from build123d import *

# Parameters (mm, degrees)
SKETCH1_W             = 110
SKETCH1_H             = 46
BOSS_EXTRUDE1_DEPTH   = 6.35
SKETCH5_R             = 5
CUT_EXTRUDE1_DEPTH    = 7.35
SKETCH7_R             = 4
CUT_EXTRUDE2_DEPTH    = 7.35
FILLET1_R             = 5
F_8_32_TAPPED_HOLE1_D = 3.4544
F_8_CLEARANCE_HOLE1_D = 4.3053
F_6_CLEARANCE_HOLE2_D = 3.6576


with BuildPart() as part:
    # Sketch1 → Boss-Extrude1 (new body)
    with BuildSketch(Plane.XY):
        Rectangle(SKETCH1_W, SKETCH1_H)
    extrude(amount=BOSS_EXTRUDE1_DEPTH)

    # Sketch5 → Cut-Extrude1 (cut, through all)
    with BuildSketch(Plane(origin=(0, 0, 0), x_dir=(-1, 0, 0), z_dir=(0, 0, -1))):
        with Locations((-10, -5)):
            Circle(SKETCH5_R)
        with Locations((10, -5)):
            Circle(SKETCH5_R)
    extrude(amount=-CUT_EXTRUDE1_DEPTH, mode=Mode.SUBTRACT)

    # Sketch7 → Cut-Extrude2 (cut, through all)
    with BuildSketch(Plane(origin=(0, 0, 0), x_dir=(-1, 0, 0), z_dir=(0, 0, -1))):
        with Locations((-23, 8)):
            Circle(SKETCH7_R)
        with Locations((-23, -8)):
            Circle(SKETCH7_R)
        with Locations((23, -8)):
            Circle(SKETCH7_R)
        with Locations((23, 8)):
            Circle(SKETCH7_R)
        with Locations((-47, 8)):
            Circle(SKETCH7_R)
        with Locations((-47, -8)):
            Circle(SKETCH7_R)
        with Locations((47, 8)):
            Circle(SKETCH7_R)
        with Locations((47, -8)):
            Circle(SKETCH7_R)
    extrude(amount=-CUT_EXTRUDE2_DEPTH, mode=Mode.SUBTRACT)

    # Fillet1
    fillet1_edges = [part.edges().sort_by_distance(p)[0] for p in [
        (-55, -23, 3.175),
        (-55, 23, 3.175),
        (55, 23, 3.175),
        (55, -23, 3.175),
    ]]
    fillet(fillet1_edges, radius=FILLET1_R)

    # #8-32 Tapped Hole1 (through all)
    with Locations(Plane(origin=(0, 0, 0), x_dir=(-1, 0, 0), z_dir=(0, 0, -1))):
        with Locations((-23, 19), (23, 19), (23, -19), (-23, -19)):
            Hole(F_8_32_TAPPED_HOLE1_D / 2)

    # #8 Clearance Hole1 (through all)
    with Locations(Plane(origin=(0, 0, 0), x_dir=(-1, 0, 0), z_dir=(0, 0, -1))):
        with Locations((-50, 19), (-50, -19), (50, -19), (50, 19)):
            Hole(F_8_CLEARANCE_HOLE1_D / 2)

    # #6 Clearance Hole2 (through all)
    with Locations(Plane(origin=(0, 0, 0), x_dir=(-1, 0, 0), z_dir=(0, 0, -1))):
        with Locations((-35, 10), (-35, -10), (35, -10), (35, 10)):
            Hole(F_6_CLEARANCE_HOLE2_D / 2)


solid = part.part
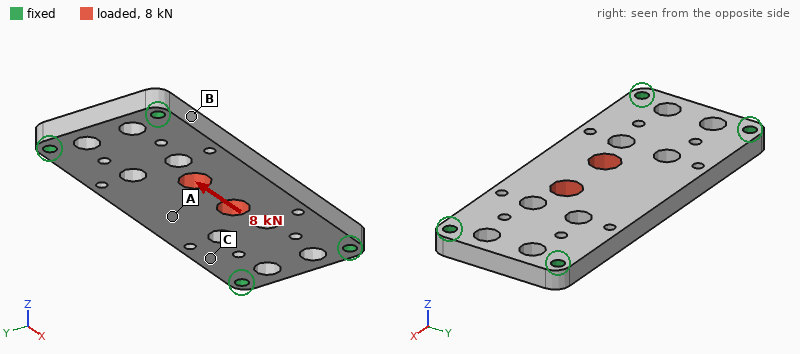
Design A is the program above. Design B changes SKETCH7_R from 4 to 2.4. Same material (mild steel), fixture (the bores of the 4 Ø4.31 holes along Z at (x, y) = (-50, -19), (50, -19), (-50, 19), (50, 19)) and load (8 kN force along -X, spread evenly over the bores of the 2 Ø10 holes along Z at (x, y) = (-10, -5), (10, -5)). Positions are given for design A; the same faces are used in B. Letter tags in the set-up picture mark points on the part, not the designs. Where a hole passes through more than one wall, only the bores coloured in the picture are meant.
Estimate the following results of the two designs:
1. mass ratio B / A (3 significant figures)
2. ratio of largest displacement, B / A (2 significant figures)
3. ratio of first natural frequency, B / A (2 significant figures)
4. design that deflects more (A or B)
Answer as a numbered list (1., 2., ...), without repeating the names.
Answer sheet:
1. 1.06
2. 0.92
3. 1.0
4. A
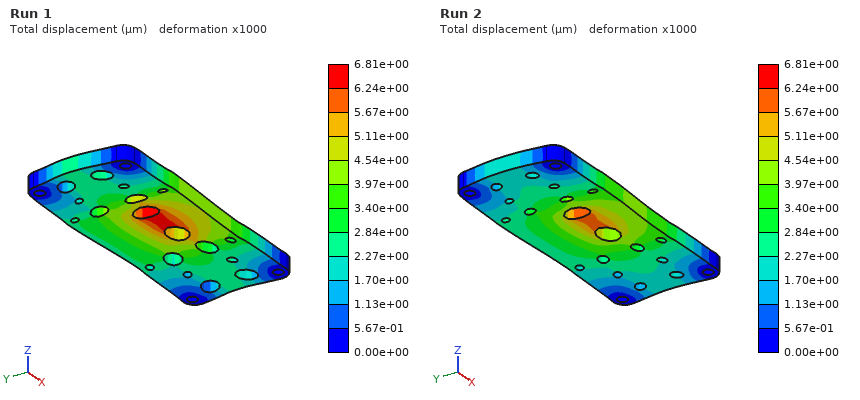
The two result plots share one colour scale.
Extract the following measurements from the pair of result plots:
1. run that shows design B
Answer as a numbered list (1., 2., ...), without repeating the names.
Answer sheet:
1. Run 2
